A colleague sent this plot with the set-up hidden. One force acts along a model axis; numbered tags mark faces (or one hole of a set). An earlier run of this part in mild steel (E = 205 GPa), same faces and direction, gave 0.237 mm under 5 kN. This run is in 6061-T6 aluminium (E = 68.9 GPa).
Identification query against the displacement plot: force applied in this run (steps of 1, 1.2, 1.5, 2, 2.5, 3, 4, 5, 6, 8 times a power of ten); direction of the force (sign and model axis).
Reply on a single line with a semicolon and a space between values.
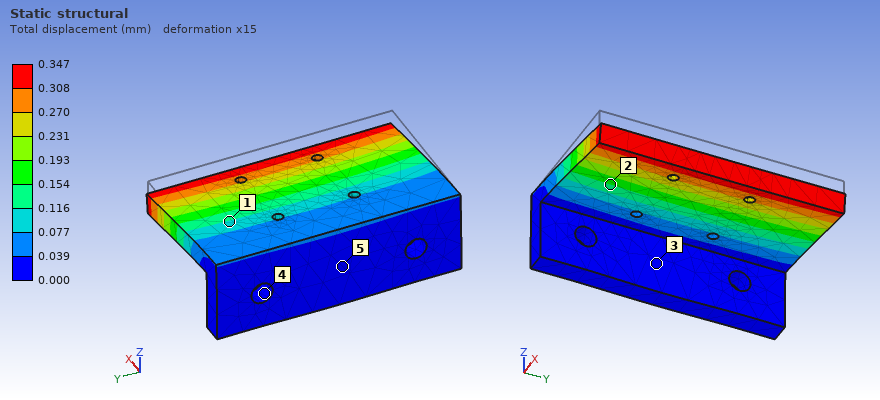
2.5 kN; -Z
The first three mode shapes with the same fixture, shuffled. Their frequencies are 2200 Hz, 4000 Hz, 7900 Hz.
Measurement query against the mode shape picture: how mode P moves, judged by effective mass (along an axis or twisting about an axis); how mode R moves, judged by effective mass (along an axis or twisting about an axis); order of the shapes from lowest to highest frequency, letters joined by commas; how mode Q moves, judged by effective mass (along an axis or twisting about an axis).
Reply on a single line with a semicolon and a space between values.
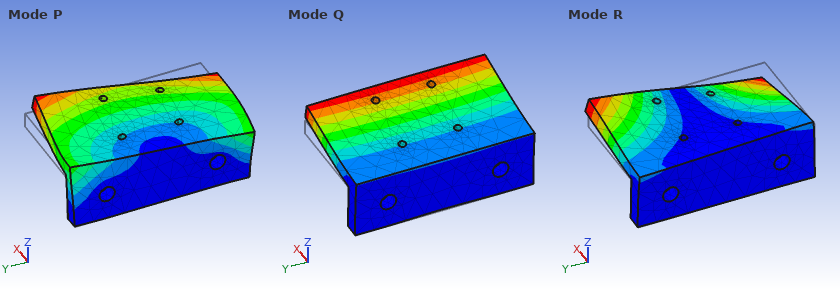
along Y; twisting about X; Q, R, P; along Z
